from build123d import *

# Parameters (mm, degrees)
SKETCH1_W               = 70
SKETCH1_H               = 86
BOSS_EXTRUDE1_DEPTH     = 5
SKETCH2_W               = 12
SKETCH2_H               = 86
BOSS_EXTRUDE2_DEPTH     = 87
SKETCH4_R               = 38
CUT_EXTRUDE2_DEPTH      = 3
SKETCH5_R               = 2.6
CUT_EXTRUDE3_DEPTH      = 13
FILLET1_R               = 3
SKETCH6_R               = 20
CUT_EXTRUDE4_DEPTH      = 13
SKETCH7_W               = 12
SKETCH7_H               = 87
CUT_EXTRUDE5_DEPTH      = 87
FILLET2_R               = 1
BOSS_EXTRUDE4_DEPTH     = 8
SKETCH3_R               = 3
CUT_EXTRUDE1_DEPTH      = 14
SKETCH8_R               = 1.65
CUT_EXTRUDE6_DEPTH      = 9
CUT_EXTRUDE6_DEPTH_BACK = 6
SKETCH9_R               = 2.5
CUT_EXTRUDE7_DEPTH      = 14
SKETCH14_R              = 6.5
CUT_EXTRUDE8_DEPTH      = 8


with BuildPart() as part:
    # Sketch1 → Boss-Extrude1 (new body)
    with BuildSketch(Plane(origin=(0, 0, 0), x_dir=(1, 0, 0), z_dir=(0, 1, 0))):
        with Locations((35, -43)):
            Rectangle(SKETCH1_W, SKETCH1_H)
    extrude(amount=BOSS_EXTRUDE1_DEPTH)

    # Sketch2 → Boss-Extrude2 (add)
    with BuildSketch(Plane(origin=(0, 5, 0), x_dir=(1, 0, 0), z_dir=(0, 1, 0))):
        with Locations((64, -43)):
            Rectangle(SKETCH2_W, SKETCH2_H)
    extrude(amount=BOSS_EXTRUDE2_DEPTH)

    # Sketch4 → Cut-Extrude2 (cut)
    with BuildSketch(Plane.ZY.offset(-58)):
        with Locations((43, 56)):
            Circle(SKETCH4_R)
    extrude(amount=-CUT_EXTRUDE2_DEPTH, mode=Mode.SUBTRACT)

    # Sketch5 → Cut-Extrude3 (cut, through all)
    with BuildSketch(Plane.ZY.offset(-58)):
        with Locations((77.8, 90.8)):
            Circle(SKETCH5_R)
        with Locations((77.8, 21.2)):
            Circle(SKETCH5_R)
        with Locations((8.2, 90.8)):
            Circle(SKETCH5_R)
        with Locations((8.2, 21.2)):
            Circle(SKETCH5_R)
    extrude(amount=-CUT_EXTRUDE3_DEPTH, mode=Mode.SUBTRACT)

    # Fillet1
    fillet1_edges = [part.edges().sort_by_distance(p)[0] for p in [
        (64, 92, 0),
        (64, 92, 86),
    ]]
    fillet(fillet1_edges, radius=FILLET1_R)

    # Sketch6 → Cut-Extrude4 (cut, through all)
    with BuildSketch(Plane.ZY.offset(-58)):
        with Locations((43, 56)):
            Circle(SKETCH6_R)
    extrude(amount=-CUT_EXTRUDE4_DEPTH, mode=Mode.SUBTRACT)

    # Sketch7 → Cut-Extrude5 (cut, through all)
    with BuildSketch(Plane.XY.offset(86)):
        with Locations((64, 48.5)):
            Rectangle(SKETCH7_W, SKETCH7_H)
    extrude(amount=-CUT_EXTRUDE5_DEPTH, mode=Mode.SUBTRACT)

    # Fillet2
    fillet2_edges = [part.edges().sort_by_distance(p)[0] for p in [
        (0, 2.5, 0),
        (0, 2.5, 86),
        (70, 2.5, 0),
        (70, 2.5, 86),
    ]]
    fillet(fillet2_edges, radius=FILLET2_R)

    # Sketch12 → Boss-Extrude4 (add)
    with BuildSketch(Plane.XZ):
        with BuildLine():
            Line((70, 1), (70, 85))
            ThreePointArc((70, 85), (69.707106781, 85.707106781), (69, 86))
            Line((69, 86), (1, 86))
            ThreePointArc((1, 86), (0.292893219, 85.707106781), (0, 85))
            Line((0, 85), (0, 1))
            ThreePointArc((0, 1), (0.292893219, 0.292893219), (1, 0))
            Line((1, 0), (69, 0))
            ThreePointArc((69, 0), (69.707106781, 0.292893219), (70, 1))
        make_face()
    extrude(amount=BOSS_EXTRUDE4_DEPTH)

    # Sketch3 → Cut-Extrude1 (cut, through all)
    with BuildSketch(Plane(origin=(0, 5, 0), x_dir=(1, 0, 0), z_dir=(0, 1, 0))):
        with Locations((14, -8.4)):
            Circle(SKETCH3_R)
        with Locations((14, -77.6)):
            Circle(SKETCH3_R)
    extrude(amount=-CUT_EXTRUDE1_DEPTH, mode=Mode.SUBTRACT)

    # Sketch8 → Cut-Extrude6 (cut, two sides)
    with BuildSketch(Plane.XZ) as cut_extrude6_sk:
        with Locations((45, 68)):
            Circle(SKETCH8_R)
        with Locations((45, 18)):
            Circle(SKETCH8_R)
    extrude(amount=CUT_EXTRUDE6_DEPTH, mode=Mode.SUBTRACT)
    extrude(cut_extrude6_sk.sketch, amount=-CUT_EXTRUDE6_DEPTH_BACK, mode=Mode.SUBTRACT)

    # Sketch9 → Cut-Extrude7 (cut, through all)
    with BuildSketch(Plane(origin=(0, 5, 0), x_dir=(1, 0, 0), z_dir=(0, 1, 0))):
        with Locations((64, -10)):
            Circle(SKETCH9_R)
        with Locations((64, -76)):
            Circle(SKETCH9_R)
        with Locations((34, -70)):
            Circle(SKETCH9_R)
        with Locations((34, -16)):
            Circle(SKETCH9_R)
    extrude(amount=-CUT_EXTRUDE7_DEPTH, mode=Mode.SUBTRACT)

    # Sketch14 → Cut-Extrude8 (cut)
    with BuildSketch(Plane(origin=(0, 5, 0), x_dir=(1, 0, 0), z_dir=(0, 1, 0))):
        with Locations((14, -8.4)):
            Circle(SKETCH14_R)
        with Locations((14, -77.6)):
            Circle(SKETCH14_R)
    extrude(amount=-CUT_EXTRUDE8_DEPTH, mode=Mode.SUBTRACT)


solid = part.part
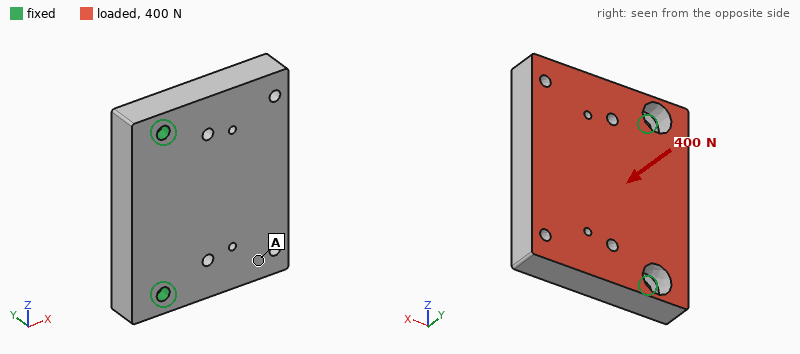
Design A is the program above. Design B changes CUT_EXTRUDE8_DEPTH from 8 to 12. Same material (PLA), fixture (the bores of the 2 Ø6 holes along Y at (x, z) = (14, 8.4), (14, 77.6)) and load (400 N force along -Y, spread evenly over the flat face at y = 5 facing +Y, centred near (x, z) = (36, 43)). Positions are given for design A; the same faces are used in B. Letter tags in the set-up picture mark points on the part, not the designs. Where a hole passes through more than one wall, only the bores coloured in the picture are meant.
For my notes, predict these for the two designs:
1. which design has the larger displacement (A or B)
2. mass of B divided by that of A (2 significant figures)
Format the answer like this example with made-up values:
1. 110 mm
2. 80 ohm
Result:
1. B
2. 0.99
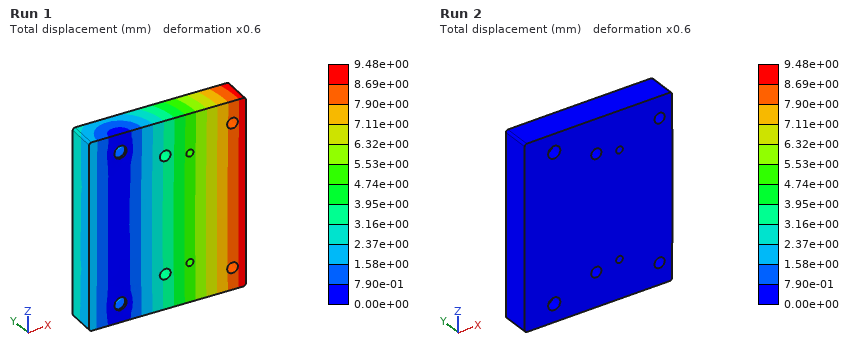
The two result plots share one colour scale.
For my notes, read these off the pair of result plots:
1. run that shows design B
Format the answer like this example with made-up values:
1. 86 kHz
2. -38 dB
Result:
1. Run 1
